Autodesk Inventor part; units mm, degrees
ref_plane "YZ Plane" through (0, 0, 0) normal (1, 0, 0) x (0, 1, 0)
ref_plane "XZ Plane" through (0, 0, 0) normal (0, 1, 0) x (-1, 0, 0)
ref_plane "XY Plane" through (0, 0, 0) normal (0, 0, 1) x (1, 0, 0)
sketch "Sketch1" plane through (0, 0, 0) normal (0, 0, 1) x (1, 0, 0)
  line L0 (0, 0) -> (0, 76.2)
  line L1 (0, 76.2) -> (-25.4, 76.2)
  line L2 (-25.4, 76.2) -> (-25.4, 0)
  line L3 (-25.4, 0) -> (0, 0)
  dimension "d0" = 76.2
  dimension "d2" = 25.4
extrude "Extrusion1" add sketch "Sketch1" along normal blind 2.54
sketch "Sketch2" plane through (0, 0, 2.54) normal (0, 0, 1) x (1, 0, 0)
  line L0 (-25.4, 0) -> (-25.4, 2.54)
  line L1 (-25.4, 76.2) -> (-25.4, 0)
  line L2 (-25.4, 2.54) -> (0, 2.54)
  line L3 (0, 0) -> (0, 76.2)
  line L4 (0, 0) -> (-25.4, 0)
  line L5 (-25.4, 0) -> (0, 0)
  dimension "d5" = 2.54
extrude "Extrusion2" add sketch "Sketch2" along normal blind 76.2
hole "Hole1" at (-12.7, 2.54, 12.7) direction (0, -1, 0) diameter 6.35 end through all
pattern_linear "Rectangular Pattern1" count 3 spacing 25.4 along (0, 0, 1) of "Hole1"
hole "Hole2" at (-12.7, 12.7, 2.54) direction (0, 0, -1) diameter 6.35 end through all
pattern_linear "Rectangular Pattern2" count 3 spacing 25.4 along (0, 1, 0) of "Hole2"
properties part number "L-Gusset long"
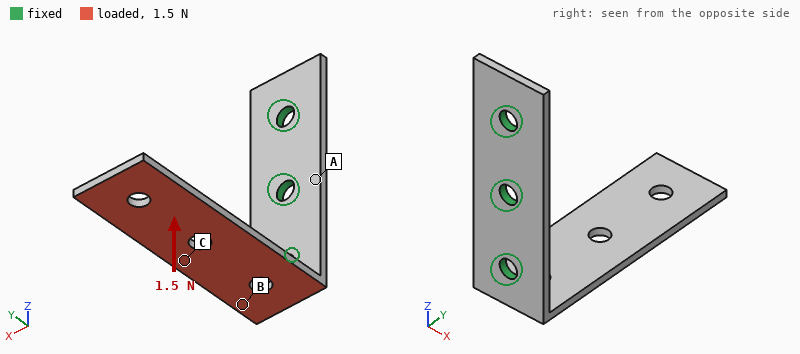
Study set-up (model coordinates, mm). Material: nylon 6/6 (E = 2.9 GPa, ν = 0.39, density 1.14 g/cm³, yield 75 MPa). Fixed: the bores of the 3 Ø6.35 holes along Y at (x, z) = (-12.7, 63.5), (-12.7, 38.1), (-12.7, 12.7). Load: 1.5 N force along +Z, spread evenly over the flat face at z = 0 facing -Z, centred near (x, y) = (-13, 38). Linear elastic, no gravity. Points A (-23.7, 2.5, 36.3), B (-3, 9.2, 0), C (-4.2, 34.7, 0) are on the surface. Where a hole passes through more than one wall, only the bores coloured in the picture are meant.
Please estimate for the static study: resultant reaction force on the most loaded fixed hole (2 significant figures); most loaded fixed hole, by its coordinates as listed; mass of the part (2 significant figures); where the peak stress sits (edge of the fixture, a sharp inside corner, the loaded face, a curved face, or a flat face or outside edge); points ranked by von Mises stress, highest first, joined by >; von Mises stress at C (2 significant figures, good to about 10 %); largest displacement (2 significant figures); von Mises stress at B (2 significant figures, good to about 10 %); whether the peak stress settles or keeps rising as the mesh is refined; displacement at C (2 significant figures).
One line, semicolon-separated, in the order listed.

1.5 N; (-12.7, 12.7); 11 g; edge of the fixture; B > C > A; 0.74 MPa; 1.2 mm; 1.8 MPa; keeps rising; 0.39 mm
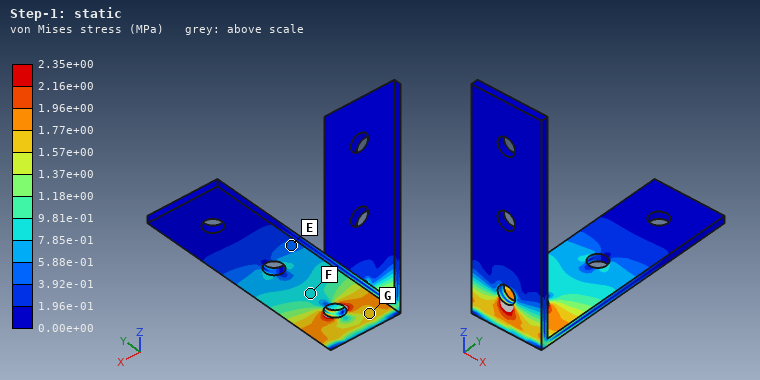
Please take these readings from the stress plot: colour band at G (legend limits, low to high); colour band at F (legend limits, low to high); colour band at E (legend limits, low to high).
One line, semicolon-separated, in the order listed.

1.57e+00 to 1.77e+00 MPa; 7.85e-01 to 9.81e-01 MPa; 3.92e-01 to 5.88e-01 MPa
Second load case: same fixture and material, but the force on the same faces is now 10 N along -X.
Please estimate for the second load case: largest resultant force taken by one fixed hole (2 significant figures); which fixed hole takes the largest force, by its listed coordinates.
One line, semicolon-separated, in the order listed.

13 N; (-12.7, 12.7)
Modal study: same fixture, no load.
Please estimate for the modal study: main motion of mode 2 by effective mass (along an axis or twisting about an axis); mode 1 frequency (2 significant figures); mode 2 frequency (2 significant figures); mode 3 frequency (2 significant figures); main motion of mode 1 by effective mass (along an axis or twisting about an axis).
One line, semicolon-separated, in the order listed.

along X; 97 Hz; 230 Hz; 610 Hz; along Z
